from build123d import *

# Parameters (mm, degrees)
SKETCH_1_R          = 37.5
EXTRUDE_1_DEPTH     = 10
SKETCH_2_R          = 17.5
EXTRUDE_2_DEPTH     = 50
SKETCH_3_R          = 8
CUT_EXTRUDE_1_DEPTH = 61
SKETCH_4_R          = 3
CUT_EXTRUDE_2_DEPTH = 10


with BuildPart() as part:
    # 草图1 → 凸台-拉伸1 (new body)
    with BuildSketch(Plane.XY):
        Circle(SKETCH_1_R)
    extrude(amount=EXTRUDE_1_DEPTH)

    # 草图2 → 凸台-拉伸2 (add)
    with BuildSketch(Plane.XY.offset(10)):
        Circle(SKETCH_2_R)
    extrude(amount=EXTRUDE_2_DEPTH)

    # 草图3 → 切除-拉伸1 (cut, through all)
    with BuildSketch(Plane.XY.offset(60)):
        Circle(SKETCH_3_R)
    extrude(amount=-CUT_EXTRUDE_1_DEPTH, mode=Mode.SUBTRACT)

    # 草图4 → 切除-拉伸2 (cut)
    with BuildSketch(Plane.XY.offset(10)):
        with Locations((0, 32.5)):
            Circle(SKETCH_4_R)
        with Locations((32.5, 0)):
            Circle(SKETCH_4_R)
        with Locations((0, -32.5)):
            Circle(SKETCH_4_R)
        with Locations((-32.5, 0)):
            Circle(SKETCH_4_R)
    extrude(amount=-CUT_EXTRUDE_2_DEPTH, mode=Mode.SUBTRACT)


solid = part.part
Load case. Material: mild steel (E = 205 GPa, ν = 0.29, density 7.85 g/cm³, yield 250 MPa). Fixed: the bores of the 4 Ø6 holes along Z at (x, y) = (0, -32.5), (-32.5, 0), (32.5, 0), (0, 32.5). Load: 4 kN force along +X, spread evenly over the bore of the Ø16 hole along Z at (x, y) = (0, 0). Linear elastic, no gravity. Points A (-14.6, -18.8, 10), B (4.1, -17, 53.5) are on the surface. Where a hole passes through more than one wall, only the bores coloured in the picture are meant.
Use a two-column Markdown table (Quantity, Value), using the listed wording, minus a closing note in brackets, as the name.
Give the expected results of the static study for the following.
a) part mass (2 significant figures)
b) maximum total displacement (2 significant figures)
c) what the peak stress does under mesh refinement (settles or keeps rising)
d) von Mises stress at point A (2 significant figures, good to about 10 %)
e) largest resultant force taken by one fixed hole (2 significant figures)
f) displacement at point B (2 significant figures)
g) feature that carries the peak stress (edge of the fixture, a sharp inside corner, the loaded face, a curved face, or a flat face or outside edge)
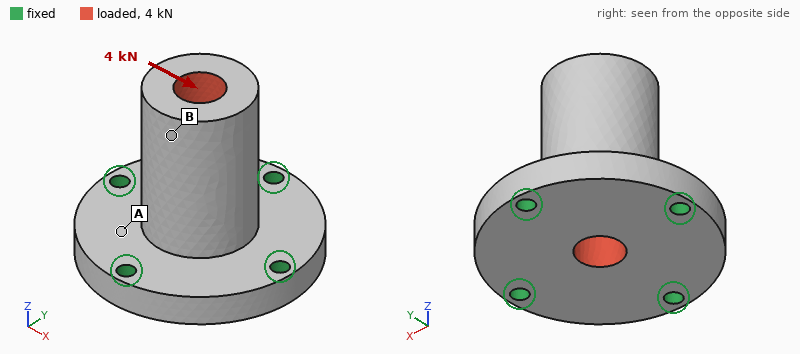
| Quantity | Value |
|---|---|
| part mass | 620 g |
| maximum total displacement | 16 µm |
| what the peak stress does under mesh refinement | keeps rising |
| von Mises stress at point A | 8.6 MPa |
| largest resultant force taken by one fixed hole | 2.2 kN |
| displacement at point B | 14 µm |
| feature that carries the peak stress | edge of the fixture |
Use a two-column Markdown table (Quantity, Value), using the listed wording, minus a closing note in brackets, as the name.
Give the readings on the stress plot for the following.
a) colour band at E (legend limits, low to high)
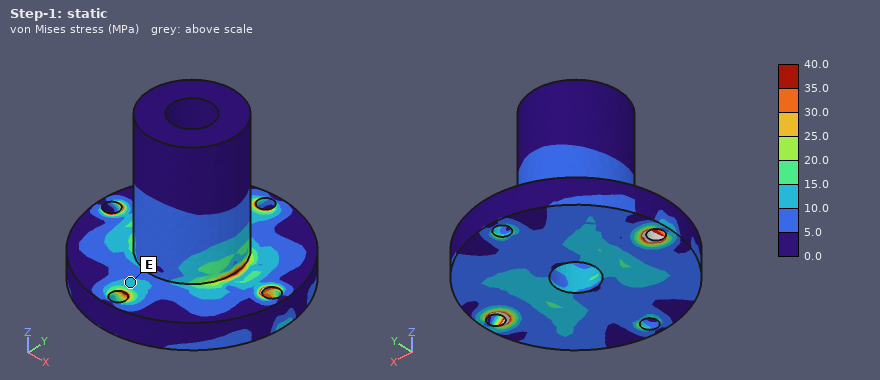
| Quantity | Value |
|---|---|
| colour band at E | 10.0 to 15.0 MPa |
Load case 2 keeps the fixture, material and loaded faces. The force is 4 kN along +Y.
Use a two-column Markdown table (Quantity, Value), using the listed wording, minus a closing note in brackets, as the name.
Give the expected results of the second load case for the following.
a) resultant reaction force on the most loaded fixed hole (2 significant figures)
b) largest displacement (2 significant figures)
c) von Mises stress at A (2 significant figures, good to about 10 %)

| Quantity | Value |
|---|---|
| resultant reaction force on the most loaded fixed hole | 2.2 kN |
| largest displacement | 16 µm |
| von Mises stress at A | 12 MPa |
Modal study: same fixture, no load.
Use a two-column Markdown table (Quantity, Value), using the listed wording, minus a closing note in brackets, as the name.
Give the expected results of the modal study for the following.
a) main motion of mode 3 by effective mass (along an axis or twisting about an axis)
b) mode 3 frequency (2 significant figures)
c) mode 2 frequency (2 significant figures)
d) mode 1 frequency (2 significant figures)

| Quantity | Value |
|---|---|
| main motion of mode 3 by effective mass | along Z |
| mode 3 frequency | 9300 Hz |
| mode 2 frequency | 4900 Hz |
| mode 1 frequency | 4900 Hz |
